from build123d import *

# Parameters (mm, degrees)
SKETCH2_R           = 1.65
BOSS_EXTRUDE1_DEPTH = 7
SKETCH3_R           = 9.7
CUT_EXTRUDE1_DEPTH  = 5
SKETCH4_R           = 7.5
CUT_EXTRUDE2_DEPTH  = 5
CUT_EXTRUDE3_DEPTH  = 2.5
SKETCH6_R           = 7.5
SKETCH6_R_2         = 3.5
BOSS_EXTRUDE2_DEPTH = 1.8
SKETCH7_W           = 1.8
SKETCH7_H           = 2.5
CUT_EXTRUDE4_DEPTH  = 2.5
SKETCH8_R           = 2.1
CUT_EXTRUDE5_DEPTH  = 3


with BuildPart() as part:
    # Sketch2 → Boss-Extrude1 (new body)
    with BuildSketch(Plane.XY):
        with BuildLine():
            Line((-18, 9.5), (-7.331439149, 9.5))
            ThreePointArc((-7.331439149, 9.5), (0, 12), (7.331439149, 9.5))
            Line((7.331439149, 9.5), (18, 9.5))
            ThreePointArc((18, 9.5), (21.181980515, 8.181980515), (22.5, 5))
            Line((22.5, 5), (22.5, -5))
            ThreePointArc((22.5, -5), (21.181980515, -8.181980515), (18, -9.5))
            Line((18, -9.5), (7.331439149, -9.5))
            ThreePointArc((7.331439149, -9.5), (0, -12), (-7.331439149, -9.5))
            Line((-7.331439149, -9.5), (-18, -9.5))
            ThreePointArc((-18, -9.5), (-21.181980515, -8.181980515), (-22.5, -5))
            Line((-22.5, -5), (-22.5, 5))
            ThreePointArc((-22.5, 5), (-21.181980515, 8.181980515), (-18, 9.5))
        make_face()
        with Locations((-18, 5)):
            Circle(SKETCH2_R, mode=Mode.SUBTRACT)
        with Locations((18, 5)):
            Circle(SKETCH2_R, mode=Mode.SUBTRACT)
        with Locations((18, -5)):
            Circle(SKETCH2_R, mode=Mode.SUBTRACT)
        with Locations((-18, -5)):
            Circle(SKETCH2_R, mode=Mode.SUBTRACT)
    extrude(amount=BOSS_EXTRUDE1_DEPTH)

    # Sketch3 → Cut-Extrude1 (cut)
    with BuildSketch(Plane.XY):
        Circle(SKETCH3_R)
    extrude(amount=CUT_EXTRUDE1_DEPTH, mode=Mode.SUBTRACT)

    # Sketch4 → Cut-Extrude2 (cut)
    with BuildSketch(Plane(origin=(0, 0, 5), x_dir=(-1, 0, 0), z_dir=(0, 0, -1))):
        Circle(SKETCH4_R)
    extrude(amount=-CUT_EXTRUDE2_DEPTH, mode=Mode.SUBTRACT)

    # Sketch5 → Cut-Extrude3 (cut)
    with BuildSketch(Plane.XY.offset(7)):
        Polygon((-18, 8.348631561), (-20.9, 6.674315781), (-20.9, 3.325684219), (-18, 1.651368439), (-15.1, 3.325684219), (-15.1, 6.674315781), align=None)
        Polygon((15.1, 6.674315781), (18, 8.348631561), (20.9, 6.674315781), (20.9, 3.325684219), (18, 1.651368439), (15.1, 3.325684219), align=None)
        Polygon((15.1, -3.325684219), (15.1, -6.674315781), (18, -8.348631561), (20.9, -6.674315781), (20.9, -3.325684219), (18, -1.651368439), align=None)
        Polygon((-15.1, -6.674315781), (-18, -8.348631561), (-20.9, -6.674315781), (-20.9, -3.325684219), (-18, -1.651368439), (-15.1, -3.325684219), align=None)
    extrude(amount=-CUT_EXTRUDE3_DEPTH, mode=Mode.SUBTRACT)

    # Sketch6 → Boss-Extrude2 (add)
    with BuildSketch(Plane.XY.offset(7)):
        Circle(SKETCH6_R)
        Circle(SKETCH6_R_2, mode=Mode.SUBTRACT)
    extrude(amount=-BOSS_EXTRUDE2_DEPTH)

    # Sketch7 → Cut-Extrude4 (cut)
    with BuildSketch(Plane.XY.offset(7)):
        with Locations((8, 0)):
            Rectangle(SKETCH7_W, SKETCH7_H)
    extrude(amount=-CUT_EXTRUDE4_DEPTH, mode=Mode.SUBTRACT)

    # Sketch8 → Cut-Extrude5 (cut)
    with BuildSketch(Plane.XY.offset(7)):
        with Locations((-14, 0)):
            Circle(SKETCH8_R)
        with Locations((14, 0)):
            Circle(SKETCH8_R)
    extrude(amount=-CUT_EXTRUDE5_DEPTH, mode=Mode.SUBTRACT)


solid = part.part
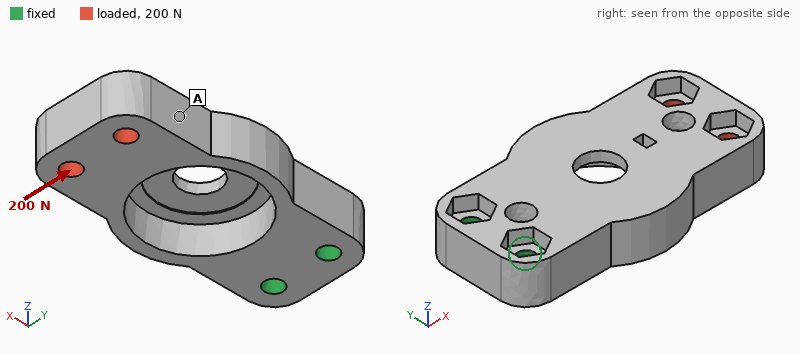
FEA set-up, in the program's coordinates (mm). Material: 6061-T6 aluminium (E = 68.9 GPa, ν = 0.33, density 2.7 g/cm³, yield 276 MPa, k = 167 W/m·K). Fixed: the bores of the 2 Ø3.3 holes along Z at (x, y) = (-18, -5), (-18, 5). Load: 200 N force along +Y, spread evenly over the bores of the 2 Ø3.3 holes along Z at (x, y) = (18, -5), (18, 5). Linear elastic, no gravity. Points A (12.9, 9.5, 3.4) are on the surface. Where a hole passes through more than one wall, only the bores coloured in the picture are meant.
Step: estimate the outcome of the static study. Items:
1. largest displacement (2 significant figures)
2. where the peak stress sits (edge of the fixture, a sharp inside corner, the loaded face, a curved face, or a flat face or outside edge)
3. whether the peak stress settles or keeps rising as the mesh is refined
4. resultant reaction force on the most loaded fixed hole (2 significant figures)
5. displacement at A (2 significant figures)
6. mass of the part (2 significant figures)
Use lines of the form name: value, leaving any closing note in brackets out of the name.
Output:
largest displacement: 47 µm
where the peak stress sits: edge of the fixture
whether the peak stress settles or keeps rising as the mesh is refined: keeps rising
resultant reaction force on the most loaded fixed hole: 580 N
displacement at A: 36 µm
mass of the part: 11 g
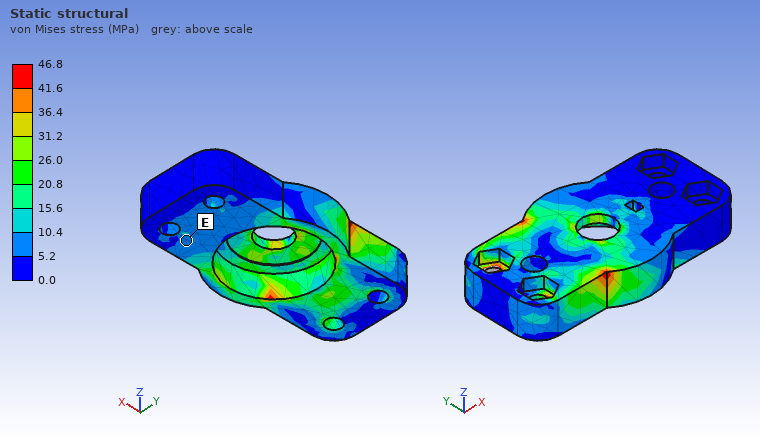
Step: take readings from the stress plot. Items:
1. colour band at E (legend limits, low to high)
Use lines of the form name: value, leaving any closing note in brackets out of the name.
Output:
colour band at E: 5.2 to 10.4 MPa
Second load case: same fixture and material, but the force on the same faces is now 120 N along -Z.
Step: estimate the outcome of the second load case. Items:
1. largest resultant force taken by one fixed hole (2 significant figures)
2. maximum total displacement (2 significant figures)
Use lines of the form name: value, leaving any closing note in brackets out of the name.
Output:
largest resultant force taken by one fixed hole: 89 N
maximum total displacement: 0.17 mm
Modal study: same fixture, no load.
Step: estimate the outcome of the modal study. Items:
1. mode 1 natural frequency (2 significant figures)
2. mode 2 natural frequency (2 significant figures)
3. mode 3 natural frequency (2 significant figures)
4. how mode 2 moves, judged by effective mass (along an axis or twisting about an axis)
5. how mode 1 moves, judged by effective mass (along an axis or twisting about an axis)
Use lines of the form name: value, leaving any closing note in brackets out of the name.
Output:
mode 1 natural frequency: 2500 Hz
mode 2 natural frequency: 5500 Hz
mode 3 natural frequency: 10 kHz
how mode 2 moves, judged by effective mass: along Y
how mode 1 moves, judged by effective mass: along Z
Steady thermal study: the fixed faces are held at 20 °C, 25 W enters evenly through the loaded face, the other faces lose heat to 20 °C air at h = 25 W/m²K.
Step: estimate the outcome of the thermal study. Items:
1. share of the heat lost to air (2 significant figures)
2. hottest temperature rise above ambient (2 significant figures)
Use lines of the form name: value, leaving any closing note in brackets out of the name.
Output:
share of the heat lost to air: 11 %
hottest temperature rise above ambient: 72 K
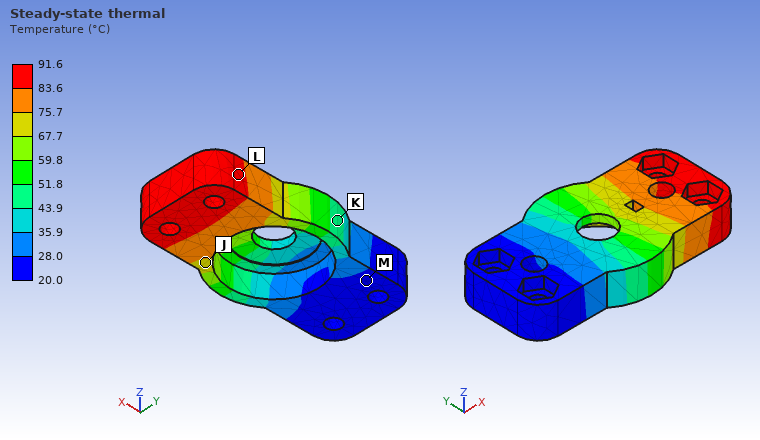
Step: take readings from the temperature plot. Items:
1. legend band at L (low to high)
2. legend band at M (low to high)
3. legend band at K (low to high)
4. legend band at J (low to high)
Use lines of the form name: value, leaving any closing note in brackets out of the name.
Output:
legend band at L: 83.6 to 91.6 °C
legend band at M: 20.0 to 28.0 °C
legend band at K: 43.9 to 51.8 °C
legend band at J: 67.7 to 75.7 °C
